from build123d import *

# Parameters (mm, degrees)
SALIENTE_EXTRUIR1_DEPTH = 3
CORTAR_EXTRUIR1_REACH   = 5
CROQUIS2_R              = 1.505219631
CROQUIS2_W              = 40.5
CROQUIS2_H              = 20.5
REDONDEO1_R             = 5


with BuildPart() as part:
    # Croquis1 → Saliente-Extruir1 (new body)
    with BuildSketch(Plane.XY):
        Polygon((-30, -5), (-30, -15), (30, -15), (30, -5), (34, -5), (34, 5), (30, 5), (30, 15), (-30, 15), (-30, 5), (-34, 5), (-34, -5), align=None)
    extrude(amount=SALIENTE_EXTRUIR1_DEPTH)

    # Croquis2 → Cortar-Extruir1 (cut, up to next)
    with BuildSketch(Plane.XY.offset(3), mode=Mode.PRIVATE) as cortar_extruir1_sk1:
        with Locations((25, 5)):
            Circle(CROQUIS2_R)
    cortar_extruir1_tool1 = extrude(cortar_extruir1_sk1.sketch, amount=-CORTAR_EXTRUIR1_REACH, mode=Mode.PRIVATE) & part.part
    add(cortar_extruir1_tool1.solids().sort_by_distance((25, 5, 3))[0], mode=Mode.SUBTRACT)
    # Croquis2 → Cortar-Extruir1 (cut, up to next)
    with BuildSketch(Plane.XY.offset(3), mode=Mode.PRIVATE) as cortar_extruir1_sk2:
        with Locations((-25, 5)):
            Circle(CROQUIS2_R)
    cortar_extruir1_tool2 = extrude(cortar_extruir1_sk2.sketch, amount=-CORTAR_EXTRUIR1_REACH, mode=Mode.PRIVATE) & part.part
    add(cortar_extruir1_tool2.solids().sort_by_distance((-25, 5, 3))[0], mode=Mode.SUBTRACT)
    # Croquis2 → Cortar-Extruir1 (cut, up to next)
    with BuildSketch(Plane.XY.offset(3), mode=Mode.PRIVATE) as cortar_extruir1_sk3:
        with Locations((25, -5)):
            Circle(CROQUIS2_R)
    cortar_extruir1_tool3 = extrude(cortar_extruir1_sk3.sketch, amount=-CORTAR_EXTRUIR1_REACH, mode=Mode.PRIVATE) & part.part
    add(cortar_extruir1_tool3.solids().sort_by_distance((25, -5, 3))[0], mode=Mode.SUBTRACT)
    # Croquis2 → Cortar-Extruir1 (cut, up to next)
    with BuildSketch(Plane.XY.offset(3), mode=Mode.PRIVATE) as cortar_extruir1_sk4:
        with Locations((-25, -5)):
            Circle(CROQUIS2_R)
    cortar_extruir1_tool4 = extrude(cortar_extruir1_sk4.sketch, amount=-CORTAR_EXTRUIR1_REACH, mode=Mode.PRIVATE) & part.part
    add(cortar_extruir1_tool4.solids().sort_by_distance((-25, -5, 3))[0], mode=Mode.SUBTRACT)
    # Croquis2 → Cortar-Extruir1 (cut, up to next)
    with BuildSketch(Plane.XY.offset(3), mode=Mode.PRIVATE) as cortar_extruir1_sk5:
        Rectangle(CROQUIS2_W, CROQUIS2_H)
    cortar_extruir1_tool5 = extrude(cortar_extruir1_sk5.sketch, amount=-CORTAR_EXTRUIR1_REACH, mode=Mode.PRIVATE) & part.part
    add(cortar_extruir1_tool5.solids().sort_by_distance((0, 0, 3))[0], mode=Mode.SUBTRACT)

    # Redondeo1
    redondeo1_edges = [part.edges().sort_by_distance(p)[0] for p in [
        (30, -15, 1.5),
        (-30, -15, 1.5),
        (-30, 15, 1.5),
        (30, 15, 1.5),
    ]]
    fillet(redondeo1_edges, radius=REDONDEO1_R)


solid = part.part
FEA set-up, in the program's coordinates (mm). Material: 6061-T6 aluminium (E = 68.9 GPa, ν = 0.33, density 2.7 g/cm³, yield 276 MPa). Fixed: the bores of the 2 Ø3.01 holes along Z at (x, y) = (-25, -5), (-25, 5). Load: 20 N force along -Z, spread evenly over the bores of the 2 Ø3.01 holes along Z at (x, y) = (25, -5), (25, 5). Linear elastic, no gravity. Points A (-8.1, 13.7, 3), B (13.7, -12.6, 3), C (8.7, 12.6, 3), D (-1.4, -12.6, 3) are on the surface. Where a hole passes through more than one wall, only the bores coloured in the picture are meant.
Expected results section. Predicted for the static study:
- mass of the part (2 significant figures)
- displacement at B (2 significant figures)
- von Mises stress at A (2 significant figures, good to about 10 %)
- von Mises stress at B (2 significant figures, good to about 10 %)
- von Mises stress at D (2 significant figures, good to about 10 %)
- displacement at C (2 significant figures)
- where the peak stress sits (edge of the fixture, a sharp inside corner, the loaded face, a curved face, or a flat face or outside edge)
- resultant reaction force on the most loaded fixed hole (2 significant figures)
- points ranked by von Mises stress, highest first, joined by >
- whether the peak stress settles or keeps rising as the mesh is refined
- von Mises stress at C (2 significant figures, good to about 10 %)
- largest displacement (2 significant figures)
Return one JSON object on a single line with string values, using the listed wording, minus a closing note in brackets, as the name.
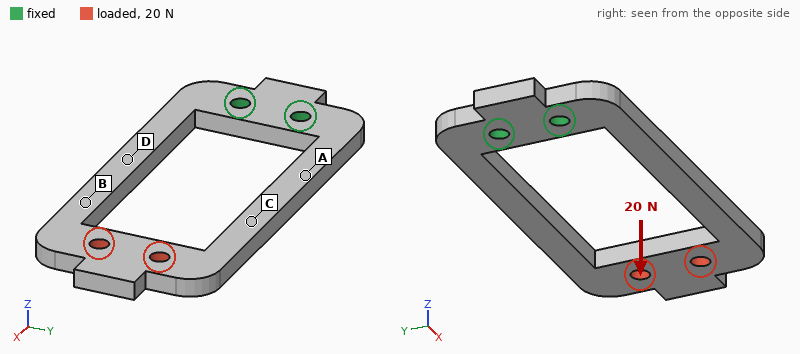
{"mass of the part": "8.1 g", "displacement at B": "0.38 mm", "von Mises stress at A": "46 MPa", "von Mises stress at B": "16 MPa", "von Mises stress at D": "37 MPa", "displacement at C": "0.31 mm", "where the peak stress sits": "a sharp inside corner", "resultant reaction force on the most loaded fixed hole": "10 N", "points ranked by von Mises stress, highest first, joined by >": "A > D > C > B", "whether the peak stress settles or keeps rising as the mesh is refined": "keeps rising", "von Mises stress at C": "23 MPa", "largest displacement": "0.73 mm"}
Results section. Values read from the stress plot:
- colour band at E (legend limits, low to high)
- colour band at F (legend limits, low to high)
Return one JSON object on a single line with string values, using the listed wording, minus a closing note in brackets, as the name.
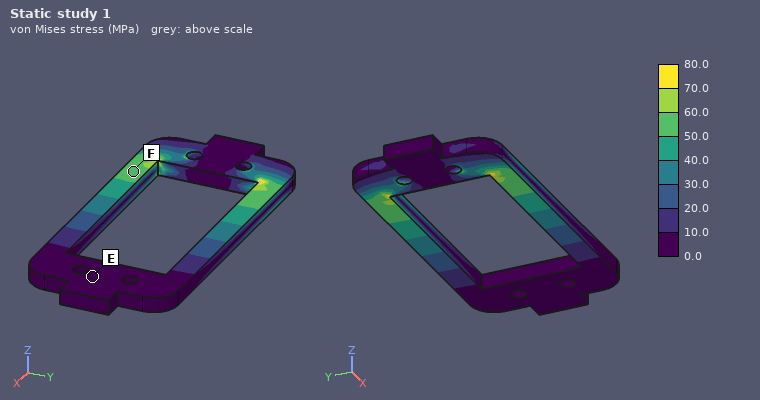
{"colour band at E": "0.0 to 10.0 MPa", "colour band at F": "50.0 to 60.0 MPa"}
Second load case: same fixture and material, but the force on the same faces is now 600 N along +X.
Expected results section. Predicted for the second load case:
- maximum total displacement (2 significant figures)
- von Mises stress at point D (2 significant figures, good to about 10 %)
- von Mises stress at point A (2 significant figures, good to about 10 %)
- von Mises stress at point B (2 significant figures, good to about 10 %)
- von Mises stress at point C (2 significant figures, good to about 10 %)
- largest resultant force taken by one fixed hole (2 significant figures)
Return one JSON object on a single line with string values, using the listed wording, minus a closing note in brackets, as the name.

{"maximum total displacement": "33 µm", "von Mises stress at point D": "21 MPa", "von Mises stress at point A": "17 MPa", "von Mises stress at point B": "21 MPa", "von Mises stress at point C": "21 MPa", "largest resultant force taken by one fixed hole": "300 N"}
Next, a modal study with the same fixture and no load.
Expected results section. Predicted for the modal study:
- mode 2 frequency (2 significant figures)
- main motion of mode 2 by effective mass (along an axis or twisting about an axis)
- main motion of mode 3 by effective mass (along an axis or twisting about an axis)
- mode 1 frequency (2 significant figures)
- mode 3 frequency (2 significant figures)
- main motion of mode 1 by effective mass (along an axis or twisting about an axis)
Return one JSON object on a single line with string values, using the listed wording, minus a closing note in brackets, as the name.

{"mode 2 frequency": "1600 Hz", "main motion of mode 2 by effective mass": "along Y", "main motion of mode 3 by effective mass": "twisting about X", "mode 1 frequency": "520 Hz", "mode 3 frequency": "1800 Hz", "main motion of mode 1 by effective mass": "along Z"}
